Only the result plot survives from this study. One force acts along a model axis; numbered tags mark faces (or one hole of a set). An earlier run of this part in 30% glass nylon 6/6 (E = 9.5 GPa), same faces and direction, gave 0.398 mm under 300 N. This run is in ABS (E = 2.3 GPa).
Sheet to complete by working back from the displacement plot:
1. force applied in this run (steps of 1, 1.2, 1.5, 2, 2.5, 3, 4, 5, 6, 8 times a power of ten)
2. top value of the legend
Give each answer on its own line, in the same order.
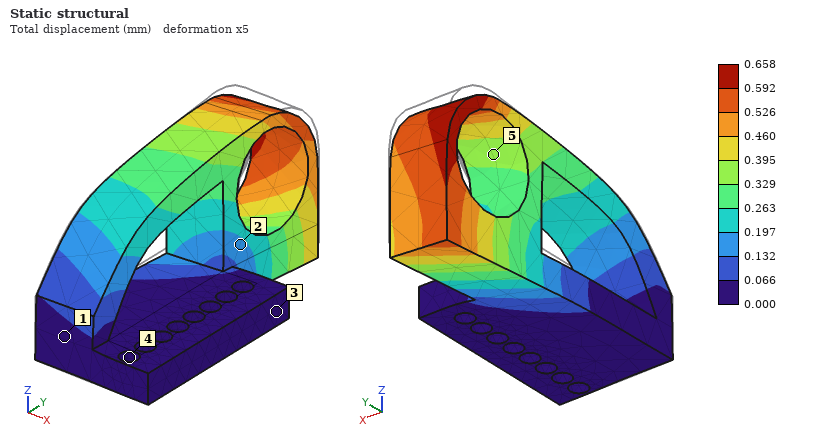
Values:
120 N
0.658 mm
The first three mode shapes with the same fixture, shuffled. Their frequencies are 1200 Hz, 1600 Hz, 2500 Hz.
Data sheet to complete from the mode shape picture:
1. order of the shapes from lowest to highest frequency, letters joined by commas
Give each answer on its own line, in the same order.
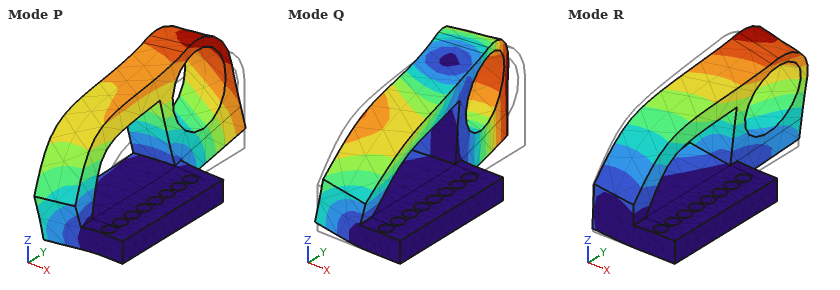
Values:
R, P, Q
